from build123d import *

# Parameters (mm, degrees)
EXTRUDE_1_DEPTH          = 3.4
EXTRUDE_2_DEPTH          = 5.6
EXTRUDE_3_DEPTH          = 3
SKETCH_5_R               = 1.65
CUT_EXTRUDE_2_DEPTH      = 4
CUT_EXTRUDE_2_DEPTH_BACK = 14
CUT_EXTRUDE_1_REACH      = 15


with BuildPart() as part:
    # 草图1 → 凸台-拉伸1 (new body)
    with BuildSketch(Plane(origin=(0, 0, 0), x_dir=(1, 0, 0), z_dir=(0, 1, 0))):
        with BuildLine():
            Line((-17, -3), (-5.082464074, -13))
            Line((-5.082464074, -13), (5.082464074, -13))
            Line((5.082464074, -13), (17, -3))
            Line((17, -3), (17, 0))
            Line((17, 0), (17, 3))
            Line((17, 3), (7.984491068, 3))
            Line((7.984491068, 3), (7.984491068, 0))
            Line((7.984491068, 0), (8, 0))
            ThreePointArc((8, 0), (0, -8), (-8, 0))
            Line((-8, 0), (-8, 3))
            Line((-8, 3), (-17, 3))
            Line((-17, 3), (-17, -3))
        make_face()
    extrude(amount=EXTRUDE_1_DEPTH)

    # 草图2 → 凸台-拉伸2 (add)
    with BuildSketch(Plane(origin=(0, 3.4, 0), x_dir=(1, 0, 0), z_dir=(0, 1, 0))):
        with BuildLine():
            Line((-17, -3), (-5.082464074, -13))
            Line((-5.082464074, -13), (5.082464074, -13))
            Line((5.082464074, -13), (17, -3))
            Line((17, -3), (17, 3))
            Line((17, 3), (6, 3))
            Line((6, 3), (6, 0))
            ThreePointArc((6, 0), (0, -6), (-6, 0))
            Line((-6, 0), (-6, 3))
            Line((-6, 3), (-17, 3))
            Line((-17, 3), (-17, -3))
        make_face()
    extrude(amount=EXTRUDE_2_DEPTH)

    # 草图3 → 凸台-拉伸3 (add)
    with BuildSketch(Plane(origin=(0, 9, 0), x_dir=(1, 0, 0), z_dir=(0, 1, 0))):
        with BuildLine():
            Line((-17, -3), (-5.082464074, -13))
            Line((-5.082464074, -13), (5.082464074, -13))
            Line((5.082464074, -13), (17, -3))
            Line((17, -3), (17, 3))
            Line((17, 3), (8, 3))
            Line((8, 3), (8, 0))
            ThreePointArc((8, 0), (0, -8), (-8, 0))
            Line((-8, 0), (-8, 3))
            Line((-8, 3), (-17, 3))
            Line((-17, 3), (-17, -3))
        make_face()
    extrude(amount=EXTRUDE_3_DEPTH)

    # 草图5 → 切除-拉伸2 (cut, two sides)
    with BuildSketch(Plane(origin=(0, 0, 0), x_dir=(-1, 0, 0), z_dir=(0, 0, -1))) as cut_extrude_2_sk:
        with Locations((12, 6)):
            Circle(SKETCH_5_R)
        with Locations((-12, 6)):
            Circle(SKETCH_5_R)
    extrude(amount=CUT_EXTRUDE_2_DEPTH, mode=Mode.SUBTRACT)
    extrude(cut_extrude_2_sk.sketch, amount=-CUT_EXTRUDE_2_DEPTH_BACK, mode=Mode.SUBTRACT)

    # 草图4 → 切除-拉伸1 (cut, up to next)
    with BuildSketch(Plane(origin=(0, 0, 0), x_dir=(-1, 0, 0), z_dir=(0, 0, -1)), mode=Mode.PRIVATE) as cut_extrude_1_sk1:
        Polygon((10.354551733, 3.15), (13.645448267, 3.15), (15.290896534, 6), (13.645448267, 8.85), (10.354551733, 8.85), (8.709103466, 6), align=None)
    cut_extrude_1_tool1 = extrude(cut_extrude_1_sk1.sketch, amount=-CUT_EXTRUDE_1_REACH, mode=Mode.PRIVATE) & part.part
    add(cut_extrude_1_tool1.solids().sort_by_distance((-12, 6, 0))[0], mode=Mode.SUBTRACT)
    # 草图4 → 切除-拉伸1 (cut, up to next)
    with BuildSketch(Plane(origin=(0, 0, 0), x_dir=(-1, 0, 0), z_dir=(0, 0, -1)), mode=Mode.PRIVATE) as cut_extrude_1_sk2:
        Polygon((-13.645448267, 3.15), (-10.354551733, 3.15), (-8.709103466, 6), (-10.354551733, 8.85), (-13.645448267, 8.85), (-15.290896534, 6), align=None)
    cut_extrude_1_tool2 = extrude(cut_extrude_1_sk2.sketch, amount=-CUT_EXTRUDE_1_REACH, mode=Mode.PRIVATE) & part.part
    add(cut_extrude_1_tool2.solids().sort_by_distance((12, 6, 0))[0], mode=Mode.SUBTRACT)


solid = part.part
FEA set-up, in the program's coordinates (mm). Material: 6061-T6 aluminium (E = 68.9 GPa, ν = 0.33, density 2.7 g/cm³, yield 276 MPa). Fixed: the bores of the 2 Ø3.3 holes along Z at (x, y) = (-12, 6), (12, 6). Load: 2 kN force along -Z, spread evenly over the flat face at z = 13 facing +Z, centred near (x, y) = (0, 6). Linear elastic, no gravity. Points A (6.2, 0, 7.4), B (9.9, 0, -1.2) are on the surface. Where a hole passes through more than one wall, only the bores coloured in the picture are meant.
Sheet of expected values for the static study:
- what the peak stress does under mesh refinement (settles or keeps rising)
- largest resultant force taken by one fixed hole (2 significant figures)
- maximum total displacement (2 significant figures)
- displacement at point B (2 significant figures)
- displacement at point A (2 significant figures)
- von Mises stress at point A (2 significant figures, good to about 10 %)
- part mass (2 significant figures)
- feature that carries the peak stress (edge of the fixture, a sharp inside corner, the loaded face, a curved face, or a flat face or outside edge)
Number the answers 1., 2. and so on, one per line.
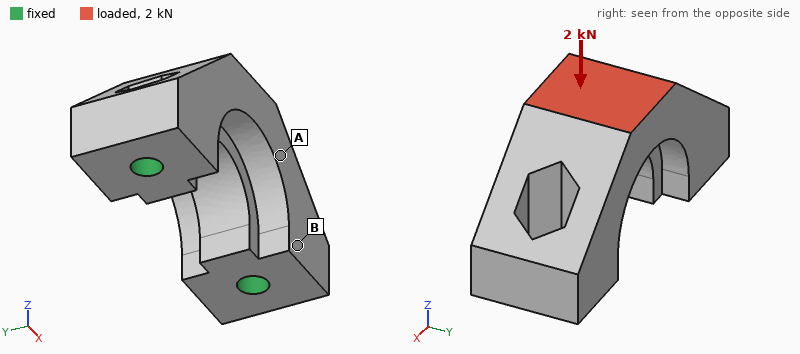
1. keeps rising
2. 1.2 kN
3. 11 µm
4. 3.9 µm
5. 6.3 µm
6. 24 MPa
7. 8.6 g
8. edge of the fixture
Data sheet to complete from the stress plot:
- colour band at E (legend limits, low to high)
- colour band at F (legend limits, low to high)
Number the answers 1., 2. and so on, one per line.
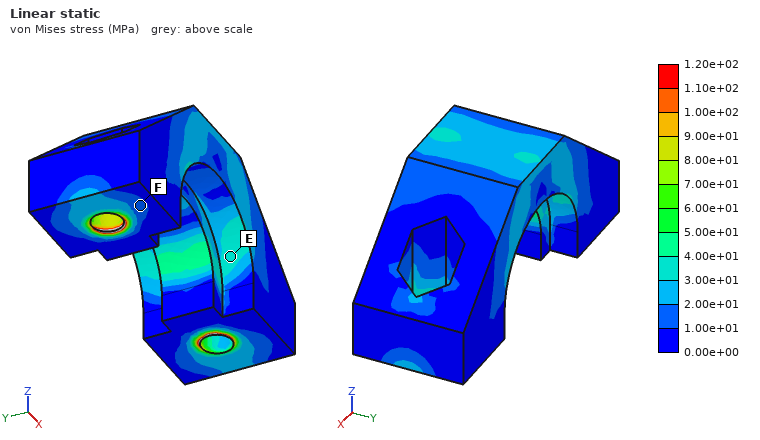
1. 3.00e+01 to 4.00e+01 MPa
2. 1.00e+01 to 2.00e+01 MPa
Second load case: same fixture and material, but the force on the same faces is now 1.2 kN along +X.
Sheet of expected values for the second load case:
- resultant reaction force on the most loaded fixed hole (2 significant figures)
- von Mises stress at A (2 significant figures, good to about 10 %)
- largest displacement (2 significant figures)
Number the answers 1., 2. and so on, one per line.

1. 890 N
2. 15 MPa
3. 9.8 µm
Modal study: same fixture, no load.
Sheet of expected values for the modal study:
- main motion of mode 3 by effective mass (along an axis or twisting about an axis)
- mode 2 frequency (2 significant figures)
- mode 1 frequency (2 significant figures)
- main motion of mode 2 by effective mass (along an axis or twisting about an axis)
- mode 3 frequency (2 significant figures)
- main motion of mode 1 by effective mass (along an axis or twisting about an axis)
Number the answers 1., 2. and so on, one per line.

1. twisting about Z
2. 26 kHz
3. 11 kHz
4. along X
5. 29 kHz
6. along Y
